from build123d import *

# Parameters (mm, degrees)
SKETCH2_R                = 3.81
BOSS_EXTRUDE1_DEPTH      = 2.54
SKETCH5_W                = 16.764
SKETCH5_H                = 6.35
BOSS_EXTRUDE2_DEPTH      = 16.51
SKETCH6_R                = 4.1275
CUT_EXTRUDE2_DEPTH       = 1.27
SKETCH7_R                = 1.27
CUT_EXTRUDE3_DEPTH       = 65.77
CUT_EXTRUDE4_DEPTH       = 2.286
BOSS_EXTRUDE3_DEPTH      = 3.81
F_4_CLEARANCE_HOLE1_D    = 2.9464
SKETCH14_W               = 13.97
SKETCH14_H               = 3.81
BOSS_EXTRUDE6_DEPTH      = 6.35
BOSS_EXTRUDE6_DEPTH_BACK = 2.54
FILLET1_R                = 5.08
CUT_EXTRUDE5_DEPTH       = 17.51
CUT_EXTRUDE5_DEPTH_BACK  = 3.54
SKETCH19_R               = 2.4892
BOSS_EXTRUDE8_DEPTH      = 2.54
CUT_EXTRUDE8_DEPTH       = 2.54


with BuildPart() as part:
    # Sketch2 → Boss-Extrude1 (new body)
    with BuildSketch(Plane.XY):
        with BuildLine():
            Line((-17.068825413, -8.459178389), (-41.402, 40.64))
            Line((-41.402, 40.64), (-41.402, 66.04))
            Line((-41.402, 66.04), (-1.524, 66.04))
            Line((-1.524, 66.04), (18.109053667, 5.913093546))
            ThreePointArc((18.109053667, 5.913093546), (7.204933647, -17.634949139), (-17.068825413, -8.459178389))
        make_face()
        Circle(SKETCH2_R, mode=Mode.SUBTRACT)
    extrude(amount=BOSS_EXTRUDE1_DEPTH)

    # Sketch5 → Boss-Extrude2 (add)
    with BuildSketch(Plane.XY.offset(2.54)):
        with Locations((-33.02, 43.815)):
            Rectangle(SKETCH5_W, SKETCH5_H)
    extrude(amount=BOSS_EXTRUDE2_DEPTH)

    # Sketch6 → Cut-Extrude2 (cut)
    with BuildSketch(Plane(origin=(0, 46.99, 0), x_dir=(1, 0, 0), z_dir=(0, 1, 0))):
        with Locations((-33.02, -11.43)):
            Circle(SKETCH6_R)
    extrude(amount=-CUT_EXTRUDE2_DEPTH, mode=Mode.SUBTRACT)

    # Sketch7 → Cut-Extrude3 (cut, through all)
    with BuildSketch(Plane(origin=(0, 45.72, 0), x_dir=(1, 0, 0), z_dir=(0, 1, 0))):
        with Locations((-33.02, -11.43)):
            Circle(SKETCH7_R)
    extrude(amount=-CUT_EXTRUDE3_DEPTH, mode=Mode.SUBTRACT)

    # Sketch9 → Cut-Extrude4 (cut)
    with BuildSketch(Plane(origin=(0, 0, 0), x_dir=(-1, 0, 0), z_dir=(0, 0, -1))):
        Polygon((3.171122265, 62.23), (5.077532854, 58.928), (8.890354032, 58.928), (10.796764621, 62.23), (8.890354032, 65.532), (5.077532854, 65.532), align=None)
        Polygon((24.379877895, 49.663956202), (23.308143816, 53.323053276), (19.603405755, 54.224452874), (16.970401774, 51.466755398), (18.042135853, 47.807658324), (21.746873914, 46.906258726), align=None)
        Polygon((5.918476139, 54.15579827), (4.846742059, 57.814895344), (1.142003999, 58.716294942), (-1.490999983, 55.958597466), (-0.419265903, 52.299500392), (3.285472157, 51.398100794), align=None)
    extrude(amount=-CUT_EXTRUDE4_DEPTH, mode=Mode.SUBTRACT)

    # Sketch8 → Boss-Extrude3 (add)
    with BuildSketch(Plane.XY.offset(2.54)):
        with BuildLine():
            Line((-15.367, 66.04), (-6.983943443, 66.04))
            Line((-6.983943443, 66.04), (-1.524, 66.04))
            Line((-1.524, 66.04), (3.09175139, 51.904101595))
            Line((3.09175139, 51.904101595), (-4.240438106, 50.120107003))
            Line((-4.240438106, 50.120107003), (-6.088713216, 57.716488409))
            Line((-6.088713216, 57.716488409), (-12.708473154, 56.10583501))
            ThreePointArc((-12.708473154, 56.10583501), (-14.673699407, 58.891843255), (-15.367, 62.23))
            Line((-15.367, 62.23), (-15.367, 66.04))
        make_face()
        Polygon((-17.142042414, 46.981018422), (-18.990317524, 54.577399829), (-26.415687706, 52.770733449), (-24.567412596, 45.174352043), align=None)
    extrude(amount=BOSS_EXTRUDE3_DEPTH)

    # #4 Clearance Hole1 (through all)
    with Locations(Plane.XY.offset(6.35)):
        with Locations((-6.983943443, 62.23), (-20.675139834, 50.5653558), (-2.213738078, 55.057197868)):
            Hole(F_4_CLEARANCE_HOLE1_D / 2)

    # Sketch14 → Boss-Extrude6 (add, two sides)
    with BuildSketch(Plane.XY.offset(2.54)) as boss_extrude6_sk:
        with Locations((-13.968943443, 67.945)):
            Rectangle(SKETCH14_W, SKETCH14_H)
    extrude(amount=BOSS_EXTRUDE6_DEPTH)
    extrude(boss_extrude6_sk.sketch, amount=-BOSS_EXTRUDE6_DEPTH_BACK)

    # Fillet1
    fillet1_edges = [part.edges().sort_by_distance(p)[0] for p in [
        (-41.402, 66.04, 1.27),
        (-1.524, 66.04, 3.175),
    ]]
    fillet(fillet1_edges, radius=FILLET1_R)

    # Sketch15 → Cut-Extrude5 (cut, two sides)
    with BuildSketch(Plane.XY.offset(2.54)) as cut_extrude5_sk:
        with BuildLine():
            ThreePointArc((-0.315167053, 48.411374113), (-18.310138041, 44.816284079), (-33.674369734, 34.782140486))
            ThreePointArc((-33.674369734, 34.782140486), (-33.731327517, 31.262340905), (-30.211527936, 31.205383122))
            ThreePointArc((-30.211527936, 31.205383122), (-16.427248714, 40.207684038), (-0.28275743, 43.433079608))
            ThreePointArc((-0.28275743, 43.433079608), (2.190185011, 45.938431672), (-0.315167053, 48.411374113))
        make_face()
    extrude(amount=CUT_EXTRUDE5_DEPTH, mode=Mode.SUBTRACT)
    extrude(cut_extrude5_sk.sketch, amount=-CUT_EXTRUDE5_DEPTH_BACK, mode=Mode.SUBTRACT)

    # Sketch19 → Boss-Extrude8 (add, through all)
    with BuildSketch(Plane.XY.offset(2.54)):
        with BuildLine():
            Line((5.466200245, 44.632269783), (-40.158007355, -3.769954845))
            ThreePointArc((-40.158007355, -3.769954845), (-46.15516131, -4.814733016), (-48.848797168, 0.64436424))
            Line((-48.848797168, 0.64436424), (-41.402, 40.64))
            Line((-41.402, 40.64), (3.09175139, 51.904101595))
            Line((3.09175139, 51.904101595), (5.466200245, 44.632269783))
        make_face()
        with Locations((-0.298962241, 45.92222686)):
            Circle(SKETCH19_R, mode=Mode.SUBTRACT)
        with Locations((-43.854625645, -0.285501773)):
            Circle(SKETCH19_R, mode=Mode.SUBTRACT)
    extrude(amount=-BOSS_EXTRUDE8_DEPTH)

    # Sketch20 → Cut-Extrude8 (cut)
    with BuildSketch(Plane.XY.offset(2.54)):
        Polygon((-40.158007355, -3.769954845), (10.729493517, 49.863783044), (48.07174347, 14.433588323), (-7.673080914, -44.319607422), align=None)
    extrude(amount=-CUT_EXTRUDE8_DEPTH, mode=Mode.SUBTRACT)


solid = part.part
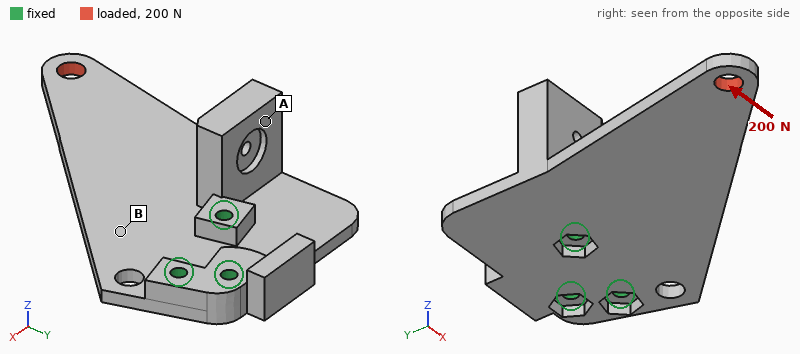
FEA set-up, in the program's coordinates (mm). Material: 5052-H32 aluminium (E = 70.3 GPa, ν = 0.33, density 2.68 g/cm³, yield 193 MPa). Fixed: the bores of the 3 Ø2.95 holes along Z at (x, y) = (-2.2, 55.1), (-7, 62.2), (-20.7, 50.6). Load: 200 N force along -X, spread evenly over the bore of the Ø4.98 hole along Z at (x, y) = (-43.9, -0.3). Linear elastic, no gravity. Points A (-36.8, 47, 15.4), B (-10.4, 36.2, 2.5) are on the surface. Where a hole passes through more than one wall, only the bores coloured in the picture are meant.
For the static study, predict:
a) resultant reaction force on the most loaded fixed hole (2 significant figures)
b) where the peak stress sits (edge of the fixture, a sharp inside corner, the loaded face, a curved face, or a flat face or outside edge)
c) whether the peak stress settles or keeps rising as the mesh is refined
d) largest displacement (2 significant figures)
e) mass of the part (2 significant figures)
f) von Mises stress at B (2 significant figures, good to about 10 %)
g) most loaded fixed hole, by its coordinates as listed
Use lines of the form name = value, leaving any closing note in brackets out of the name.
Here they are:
resultant reaction force on the most loaded fixed hole = 460 N
where the peak stress sits = edge of the fixture
whether the peak stress settles or keeps rising as the mesh is refined = keeps rising
largest displacement = 65 µm
mass of the part = 22 g
von Mises stress at B = 12 MPa
most loaded fixed hole, by its coordinates as listed = (-20.7, 50.6)
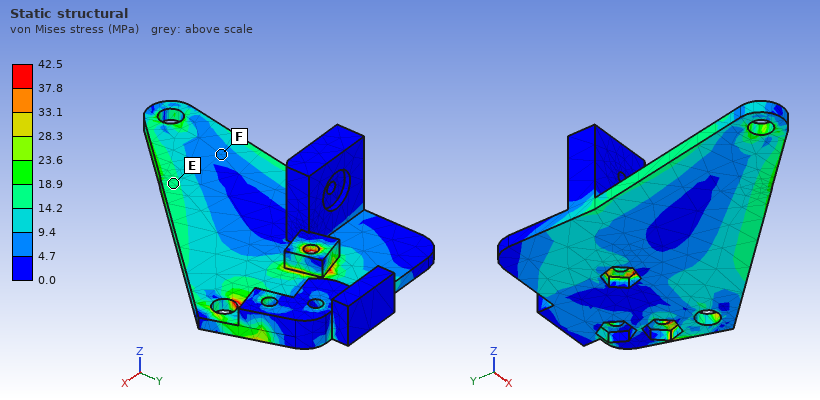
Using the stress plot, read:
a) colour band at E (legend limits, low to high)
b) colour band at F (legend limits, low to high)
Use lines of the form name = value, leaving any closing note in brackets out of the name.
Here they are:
colour band at E = 14.2 to 18.9 MPa
colour band at F = 4.7 to 9.4 MPa
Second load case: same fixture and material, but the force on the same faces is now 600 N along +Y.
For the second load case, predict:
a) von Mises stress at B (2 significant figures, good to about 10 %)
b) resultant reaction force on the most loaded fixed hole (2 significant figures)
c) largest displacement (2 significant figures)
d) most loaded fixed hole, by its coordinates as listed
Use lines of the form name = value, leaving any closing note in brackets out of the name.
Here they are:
von Mises stress at B = 14 MPa
resultant reaction force on the most loaded fixed hole = 970 N
largest displacement = 0.13 mm
most loaded fixed hole, by its coordinates as listed = (-20.7, 50.6)
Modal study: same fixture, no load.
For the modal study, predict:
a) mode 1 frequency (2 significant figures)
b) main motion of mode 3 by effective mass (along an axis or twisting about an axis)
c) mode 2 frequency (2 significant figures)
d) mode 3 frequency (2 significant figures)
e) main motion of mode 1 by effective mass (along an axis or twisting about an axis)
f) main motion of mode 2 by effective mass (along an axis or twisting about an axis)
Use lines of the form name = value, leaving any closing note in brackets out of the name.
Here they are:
mode 1 frequency = 1100 Hz
main motion of mode 3 by effective mass = along Z
mode 2 frequency = 3700 Hz
mode 3 frequency = 4100 Hz
main motion of mode 1 by effective mass = along Z
main motion of mode 2 by effective mass = twisting about Y
